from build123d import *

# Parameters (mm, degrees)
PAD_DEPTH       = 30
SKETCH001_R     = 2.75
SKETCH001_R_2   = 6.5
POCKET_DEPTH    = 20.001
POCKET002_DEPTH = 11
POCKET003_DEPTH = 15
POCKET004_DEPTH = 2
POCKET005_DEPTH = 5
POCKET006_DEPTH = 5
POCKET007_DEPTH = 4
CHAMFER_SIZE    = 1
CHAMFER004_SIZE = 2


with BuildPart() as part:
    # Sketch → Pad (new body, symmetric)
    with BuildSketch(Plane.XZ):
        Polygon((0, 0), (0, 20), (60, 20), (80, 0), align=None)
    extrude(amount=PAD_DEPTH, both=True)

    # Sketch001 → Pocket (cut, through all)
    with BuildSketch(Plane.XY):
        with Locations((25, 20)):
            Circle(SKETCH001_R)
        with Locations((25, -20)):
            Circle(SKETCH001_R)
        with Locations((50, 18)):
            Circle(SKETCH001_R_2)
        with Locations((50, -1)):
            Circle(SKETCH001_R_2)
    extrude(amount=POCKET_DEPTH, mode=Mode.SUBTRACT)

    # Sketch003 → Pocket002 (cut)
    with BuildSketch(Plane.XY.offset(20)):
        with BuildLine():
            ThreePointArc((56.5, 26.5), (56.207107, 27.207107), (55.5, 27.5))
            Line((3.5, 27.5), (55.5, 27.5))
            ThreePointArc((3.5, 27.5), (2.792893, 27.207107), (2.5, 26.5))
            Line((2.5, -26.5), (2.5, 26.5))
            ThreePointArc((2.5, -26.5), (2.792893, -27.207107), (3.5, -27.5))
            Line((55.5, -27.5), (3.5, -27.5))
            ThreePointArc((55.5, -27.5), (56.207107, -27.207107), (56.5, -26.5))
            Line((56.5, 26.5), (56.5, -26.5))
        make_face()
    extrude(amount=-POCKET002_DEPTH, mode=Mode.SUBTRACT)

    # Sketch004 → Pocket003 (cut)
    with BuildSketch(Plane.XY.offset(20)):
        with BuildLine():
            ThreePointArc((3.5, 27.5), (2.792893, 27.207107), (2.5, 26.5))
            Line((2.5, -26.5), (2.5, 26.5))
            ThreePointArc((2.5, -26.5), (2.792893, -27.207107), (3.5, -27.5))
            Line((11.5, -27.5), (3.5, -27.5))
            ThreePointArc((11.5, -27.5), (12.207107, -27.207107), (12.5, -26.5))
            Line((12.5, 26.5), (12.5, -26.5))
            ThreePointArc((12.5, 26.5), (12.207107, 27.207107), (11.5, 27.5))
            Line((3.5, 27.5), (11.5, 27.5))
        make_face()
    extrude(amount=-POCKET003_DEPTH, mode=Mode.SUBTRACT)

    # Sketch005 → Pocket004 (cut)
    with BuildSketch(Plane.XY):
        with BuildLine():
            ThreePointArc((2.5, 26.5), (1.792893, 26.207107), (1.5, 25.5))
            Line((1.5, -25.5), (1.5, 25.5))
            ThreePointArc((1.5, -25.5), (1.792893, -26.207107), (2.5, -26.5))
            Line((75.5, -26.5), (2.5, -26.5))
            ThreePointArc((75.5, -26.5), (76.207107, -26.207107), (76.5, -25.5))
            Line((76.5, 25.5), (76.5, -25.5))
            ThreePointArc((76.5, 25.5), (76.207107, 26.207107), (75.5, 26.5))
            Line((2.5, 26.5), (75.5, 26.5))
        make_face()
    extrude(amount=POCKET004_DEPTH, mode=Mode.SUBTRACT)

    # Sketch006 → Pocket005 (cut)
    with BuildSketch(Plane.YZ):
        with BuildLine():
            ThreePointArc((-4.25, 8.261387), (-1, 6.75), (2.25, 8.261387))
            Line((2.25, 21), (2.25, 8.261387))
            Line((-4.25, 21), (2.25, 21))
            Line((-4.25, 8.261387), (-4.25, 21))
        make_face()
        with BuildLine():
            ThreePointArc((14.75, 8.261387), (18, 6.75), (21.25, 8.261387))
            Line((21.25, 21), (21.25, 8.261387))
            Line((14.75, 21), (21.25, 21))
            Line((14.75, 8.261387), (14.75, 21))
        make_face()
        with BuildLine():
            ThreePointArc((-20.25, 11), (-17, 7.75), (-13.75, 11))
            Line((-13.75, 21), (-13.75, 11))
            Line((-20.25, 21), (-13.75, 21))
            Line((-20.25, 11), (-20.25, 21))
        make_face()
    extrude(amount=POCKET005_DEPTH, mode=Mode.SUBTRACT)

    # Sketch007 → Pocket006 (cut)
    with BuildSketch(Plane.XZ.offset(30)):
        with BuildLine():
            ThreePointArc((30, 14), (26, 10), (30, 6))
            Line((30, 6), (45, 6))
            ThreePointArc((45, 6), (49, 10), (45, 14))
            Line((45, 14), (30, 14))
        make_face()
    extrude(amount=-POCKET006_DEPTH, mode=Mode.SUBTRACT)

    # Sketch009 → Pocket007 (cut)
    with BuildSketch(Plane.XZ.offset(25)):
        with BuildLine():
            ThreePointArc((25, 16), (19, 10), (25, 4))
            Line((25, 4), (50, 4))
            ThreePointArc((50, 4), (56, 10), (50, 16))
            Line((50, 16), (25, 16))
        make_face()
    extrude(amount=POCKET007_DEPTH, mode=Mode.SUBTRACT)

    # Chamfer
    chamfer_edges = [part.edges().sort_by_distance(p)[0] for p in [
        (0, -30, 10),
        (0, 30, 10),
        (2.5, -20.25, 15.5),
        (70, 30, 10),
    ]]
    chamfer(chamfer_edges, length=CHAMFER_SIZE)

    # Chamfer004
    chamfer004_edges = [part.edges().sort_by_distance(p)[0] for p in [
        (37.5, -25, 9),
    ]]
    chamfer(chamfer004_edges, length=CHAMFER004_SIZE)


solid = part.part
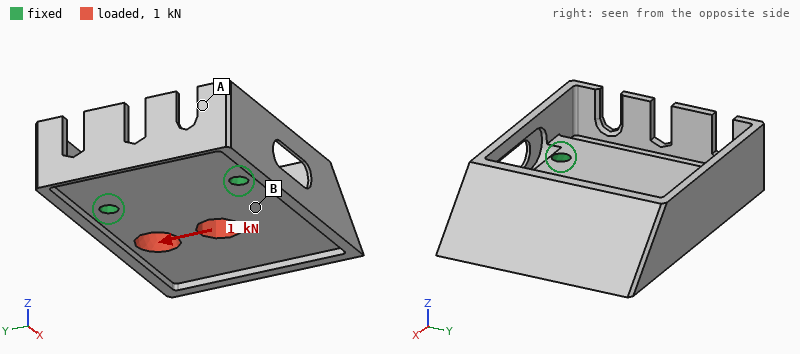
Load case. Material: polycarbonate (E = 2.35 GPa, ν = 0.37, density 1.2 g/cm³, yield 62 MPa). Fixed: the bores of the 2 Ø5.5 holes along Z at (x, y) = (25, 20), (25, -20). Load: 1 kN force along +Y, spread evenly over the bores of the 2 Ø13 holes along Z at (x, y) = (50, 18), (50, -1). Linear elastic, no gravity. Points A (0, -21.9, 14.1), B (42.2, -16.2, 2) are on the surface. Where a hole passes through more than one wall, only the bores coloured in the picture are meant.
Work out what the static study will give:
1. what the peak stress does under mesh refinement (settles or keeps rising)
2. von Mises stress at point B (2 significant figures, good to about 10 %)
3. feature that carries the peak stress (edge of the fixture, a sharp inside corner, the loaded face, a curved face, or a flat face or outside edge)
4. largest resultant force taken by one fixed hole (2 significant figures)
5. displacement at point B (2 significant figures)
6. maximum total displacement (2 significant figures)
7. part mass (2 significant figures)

keeps rising
4.3 MPa
edge of the fixture
790 N
0.074 mm
0.22 mm
44 g
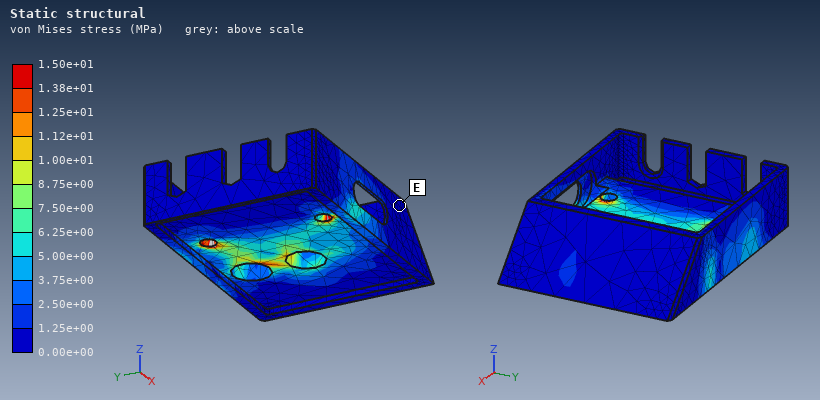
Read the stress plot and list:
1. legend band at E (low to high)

0.00e+00 to 1.25e+00 MPa
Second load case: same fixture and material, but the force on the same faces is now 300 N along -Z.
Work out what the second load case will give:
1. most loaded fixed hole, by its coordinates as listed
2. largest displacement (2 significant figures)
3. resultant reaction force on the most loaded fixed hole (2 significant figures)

(25, 20)
0.86 mm
210 N
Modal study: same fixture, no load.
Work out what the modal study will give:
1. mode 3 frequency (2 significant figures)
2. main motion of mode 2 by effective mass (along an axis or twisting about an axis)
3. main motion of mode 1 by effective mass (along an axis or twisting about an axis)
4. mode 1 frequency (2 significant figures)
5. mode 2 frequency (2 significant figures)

1600 Hz
twisting about X
along Z
590 Hz
1100 Hz
